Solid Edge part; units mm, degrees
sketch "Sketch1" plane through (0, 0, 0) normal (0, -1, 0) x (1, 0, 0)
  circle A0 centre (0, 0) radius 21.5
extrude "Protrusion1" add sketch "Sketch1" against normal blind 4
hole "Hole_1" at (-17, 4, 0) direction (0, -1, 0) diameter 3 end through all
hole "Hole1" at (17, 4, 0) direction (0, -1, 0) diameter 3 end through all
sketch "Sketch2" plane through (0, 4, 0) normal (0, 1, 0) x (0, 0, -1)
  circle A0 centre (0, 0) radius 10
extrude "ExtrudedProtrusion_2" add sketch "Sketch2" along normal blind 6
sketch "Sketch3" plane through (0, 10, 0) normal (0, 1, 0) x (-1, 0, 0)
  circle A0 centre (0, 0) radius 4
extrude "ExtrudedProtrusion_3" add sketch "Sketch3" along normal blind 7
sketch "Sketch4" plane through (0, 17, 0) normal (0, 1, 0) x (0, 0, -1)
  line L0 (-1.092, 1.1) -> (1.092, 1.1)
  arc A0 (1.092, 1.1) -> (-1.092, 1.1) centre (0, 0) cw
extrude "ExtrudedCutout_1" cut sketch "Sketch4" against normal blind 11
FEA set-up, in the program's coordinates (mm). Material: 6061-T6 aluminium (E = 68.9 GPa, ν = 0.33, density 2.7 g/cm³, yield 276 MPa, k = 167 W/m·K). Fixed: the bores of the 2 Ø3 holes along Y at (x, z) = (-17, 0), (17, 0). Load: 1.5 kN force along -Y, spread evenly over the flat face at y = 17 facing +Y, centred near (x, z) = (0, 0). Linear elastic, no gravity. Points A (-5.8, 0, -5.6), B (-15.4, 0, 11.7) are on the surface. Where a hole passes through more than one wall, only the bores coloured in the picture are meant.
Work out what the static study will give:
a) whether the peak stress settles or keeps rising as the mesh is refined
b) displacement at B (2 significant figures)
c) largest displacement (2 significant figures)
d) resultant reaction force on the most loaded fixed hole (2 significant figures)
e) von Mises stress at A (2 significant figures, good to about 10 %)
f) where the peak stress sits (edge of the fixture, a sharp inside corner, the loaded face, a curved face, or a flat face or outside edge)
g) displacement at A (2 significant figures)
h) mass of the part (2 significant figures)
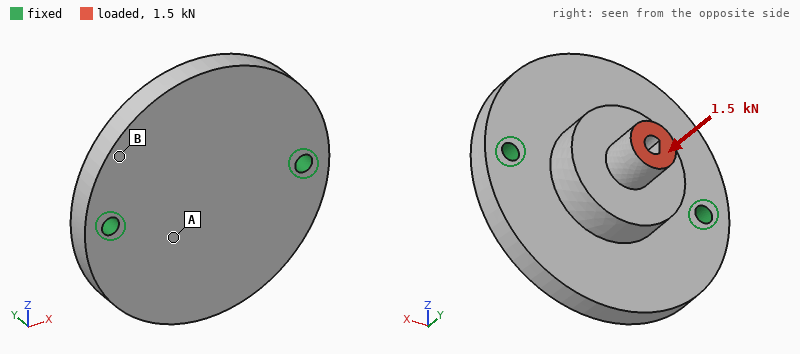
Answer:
keeps rising
8.8 µm
22 µm
810 N
21 MPa
edge of the fixture
17 µm
21 g
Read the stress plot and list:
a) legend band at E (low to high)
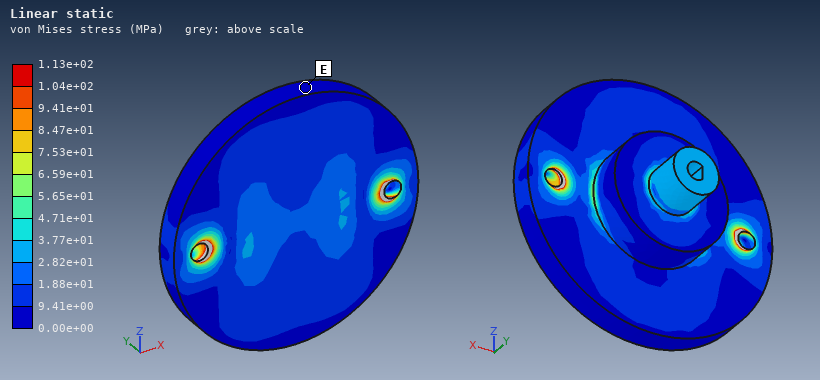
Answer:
0.00e+00 to 9.41e+00 MPa
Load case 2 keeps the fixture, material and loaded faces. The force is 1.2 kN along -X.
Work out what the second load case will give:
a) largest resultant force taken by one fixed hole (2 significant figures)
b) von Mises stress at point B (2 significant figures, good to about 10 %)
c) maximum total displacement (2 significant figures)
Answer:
880 N
13 MPa
52 µm
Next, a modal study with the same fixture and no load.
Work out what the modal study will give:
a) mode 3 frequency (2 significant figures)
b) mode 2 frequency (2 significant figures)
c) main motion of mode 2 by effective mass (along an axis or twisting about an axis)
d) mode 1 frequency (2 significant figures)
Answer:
19 kHz
10 kHz
along Y
5600 Hz
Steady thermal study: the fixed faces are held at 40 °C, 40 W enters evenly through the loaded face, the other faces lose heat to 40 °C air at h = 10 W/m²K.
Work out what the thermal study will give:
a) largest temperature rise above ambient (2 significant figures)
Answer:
69 K
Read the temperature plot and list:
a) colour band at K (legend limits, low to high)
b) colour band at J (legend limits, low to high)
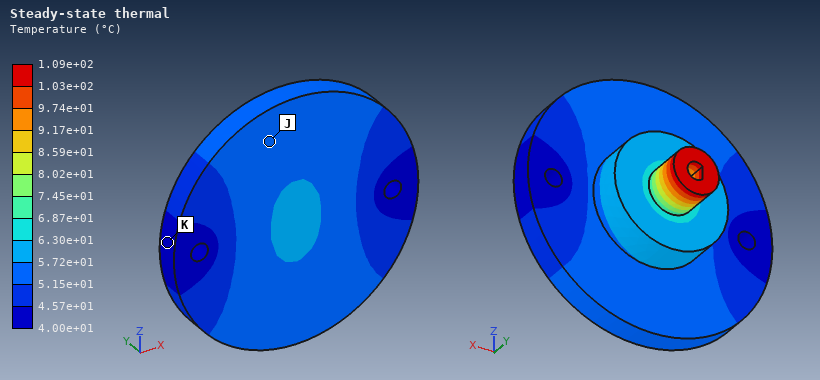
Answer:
4.00e+01 to 4.57e+01 °C
5.15e+01 to 5.72e+01 °C
